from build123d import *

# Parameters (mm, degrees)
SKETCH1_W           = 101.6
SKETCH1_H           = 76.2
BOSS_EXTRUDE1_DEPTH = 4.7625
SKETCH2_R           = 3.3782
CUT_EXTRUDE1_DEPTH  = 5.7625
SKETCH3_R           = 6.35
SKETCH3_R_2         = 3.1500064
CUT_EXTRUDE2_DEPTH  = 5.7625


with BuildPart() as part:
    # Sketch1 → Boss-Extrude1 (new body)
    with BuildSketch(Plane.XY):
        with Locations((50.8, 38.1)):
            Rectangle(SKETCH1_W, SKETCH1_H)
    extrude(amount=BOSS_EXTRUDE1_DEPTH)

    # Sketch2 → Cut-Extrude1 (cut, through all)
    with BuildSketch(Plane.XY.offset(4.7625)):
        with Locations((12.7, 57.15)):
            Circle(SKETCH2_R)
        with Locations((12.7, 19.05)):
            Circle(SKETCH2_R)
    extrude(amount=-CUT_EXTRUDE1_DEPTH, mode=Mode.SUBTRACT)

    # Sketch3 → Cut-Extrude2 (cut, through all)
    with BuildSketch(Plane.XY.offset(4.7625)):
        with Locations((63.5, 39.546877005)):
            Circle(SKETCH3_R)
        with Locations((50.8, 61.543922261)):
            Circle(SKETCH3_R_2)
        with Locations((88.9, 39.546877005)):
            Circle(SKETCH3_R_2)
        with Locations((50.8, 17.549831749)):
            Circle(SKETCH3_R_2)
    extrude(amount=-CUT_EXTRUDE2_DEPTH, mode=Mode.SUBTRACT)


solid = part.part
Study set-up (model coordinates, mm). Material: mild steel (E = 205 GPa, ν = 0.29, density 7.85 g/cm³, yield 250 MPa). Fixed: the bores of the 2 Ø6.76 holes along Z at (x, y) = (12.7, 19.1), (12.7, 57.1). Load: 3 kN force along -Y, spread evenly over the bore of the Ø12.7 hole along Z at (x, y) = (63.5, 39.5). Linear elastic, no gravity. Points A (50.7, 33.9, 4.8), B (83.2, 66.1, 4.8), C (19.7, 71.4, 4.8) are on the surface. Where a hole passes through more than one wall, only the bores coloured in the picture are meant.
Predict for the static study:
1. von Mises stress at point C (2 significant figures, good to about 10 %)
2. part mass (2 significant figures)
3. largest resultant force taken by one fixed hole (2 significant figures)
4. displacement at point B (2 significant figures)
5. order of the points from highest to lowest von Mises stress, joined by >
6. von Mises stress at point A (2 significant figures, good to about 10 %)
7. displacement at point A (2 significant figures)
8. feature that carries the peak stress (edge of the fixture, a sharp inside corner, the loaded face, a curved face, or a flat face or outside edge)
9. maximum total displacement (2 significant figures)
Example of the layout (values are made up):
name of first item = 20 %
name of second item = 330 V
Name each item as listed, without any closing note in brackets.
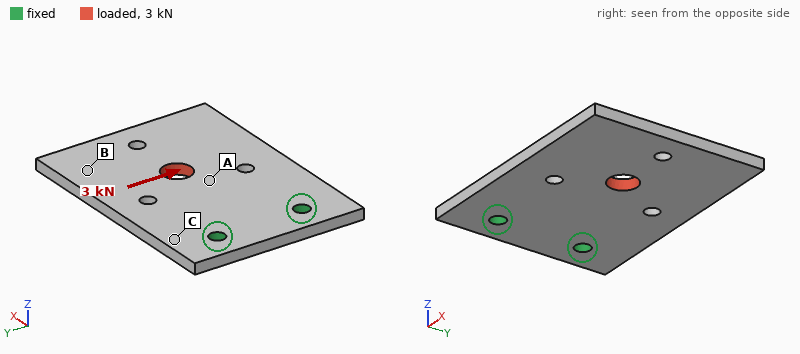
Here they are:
von Mises stress at point C = 14 MPa
part mass = 280 g
largest resultant force taken by one fixed hole = 3.8 kN
displacement at point B = 20 µm
order of the points from highest to lowest von Mises stress, joined by > = A > C > B
von Mises stress at point A = 25 MPa
displacement at point A = 11 µm
feature that carries the peak stress = edge of the fixture
maximum total displacement = 24 µm
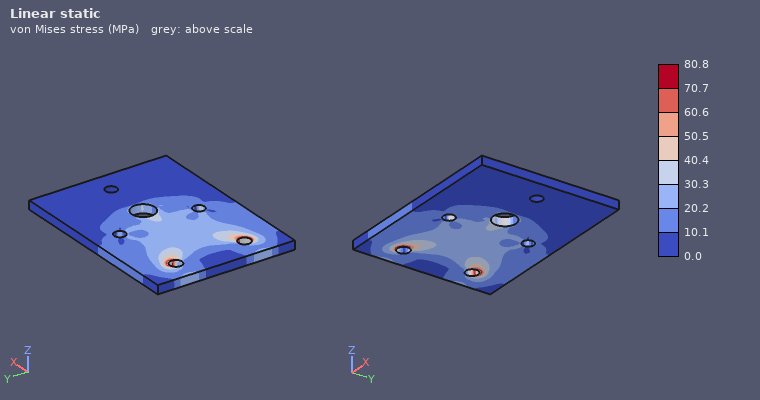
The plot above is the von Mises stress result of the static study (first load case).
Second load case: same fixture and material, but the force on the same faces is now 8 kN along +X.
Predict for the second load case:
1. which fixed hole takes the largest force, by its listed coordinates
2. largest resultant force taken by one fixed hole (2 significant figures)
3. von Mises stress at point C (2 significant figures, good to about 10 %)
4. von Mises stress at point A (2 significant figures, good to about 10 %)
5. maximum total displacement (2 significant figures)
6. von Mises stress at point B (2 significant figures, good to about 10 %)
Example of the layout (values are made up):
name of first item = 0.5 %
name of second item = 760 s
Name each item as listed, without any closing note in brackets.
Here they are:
which fixed hole takes the largest force, by its listed coordinates = (12.7, 57.1)
largest resultant force taken by one fixed hole = 4.3 kN
von Mises stress at point C = 11 MPa
von Mises stress at point A = 40 MPa
maximum total displacement = 11 µm
von Mises stress at point B = 8.2 MPa
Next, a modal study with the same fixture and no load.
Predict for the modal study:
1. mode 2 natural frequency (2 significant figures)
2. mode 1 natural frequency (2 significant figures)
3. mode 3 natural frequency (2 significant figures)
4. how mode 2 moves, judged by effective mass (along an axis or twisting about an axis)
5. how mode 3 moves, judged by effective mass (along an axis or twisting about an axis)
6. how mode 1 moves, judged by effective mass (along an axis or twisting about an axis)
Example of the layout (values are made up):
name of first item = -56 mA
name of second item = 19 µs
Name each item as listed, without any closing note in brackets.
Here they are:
mode 2 natural frequency = 1300 Hz
mode 1 natural frequency = 500 Hz
mode 3 natural frequency = 3000 Hz
how mode 2 moves, judged by effective mass = twisting about X
how mode 3 moves, judged by effective mass = along Z
how mode 1 moves, judged by effective mass = along Z
